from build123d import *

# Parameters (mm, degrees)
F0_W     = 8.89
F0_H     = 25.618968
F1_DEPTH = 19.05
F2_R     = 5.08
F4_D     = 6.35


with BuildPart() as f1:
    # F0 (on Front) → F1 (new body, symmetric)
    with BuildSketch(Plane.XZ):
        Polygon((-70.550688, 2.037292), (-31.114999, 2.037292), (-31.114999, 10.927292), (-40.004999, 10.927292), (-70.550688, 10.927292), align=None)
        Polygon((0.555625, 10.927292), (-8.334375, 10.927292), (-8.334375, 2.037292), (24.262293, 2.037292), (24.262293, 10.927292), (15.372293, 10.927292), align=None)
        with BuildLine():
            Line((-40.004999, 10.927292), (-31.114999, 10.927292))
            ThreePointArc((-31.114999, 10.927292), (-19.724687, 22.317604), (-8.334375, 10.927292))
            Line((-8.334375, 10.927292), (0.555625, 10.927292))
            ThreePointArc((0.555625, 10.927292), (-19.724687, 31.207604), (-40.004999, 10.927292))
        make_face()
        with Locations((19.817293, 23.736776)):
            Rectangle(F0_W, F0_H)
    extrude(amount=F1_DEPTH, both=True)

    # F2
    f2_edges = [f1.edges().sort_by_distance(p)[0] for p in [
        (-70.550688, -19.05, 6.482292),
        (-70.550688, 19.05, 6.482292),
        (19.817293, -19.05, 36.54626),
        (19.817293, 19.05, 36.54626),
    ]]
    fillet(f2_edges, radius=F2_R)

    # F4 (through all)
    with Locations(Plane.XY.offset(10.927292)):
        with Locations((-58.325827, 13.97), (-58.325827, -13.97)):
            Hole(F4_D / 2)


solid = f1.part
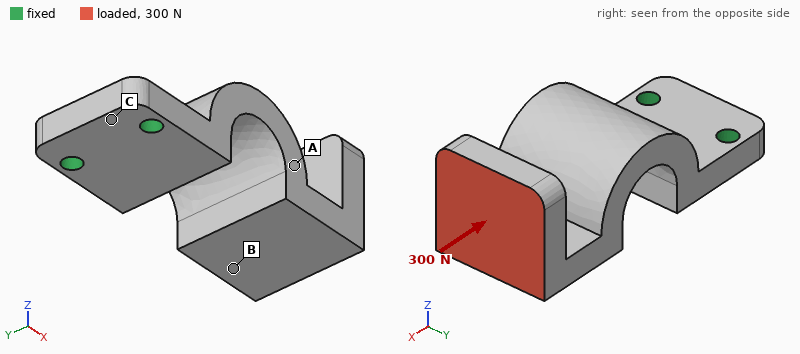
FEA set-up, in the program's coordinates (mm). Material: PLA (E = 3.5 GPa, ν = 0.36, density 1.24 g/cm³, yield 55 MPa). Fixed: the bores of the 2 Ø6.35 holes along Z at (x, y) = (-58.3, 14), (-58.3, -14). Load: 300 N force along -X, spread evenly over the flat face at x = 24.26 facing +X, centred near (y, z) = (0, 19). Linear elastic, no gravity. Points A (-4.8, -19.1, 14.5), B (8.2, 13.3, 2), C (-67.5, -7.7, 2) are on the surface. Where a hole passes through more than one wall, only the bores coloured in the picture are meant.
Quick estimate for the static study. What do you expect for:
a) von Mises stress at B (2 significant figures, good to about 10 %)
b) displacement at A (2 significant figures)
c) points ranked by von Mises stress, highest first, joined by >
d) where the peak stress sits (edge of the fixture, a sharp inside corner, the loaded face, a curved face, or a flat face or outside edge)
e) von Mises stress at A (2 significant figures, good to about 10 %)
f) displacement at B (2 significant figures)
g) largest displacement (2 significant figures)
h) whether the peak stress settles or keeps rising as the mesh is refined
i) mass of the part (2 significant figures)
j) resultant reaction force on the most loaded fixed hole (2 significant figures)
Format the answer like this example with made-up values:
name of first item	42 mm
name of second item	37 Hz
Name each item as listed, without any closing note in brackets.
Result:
von Mises stress at B	6.5 MPa
displacement at A	0.43 mm
points ranked by von Mises stress, highest first, joined by >	B > A > C
where the peak stress sits	edge of the fixture
von Mises stress at A	2.6 MPa
displacement at B	0.53 mm
largest displacement	1.1 mm
whether the peak stress settles or keeps rising as the mesh is refined	keeps rising
mass of the part	61 g
resultant reaction force on the most loaded fixed hole	150 N
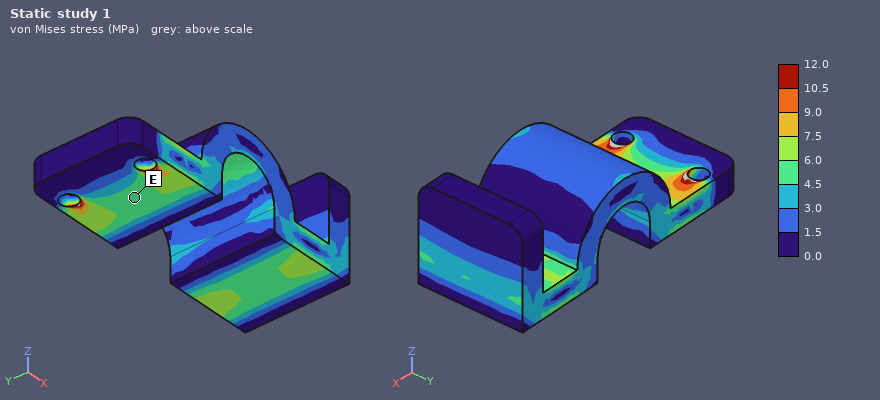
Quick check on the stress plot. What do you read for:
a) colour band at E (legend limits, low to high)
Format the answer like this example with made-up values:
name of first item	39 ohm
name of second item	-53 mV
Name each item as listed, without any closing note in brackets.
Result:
colour band at E	4.5 to 6.0 MPa
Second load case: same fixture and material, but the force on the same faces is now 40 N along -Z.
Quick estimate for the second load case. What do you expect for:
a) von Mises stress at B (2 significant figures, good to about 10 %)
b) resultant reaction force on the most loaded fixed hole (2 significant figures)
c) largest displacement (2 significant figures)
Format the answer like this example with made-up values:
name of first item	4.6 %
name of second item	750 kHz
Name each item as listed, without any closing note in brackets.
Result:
von Mises stress at B	1.3 MPa
resultant reaction force on the most loaded fixed hole	22 N
largest displacement	1.2 mm
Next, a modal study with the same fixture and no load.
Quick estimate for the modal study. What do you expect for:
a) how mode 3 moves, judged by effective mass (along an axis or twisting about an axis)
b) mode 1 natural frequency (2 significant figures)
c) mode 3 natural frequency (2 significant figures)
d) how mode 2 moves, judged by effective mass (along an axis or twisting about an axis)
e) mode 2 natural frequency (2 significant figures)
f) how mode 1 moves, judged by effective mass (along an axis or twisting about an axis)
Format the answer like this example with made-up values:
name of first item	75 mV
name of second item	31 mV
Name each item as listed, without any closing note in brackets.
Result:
how mode 3 moves, judged by effective mass	along X
mode 1 natural frequency	210 Hz
mode 3 natural frequency	900 Hz
how mode 2 moves, judged by effective mass	along Y
mode 2 natural frequency	480 Hz
how mode 1 moves, judged by effective mass	along Z
